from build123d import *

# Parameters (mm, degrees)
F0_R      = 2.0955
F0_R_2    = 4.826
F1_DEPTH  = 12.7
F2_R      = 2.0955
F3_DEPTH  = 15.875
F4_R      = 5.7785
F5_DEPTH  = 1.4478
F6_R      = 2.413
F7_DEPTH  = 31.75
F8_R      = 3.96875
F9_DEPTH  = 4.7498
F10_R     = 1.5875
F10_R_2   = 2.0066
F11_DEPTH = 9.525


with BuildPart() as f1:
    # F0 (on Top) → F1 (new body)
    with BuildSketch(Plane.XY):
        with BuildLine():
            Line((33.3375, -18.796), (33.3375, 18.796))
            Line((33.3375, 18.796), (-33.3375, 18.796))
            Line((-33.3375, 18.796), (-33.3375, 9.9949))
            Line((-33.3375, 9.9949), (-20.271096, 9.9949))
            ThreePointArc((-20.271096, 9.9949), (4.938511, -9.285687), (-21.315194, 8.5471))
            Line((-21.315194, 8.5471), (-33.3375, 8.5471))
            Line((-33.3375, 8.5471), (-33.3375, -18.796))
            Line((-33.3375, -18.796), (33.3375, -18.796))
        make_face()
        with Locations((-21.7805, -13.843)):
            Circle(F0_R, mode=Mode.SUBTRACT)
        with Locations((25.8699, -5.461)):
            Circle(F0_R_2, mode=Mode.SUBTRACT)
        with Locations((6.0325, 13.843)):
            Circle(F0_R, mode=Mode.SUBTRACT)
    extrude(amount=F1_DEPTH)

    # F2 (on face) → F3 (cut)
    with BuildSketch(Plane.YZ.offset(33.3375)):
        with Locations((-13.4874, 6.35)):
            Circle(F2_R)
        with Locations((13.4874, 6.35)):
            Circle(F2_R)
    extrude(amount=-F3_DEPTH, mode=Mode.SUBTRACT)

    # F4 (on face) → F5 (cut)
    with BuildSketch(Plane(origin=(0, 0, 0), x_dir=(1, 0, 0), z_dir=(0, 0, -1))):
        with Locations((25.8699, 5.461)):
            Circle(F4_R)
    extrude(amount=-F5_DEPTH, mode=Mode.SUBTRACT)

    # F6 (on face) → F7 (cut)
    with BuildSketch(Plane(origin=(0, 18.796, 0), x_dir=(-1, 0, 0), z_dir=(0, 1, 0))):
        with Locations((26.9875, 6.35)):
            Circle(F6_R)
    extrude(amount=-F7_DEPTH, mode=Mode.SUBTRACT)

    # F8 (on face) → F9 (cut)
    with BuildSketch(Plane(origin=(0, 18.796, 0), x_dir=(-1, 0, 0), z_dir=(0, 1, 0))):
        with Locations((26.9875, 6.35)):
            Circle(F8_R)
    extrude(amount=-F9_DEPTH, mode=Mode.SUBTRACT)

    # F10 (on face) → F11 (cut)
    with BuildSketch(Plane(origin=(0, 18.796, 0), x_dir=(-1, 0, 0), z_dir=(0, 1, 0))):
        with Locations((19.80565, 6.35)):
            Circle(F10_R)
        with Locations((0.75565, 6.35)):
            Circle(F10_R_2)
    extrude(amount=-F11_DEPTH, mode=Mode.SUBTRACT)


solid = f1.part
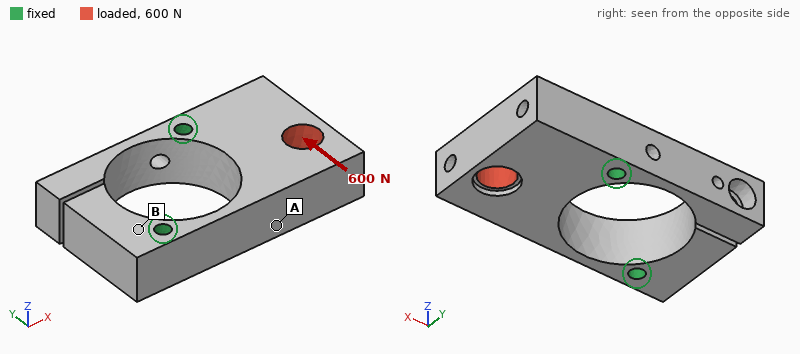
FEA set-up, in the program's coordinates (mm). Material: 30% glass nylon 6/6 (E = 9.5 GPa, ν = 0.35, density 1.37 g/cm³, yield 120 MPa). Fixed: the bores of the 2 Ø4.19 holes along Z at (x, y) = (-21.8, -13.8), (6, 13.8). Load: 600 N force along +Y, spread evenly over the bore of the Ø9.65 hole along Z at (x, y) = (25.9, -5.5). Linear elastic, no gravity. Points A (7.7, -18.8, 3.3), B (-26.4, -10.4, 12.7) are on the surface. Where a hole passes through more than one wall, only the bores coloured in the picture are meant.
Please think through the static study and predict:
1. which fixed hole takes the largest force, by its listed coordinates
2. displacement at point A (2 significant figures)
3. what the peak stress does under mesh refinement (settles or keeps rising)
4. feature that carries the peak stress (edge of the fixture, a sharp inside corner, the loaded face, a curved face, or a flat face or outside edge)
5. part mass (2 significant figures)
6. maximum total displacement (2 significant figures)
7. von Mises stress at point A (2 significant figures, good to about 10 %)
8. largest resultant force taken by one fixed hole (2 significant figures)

(6, 13.8)
27 µm
keeps rising
edge of the fixture
26 g
56 µm
6.6 MPa
670 N
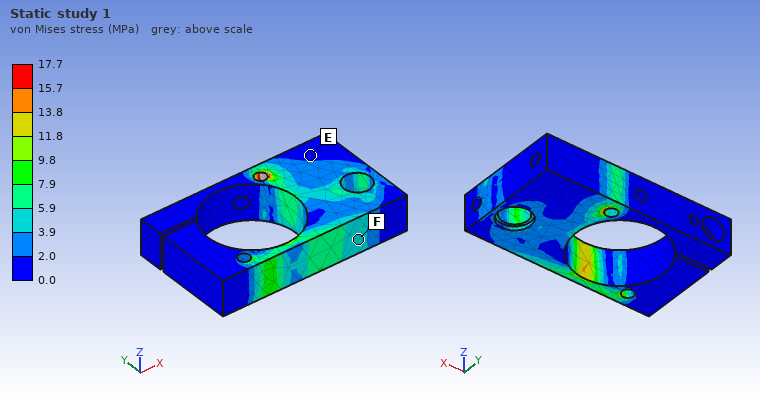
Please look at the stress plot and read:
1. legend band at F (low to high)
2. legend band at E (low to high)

3.9 to 5.9 MPa
0.0 to 2.0 MPa
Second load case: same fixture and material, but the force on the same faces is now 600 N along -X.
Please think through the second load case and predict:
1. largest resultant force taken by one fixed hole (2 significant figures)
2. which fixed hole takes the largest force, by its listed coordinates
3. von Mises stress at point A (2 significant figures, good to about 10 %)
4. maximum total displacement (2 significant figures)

330 N
(-21.8, -13.8)
6.8 MPa
40 µm
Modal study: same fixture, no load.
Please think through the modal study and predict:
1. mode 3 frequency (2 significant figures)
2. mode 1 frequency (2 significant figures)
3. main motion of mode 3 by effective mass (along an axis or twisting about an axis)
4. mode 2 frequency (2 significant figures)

3000 Hz
830 Hz
along Z
2300 Hz
